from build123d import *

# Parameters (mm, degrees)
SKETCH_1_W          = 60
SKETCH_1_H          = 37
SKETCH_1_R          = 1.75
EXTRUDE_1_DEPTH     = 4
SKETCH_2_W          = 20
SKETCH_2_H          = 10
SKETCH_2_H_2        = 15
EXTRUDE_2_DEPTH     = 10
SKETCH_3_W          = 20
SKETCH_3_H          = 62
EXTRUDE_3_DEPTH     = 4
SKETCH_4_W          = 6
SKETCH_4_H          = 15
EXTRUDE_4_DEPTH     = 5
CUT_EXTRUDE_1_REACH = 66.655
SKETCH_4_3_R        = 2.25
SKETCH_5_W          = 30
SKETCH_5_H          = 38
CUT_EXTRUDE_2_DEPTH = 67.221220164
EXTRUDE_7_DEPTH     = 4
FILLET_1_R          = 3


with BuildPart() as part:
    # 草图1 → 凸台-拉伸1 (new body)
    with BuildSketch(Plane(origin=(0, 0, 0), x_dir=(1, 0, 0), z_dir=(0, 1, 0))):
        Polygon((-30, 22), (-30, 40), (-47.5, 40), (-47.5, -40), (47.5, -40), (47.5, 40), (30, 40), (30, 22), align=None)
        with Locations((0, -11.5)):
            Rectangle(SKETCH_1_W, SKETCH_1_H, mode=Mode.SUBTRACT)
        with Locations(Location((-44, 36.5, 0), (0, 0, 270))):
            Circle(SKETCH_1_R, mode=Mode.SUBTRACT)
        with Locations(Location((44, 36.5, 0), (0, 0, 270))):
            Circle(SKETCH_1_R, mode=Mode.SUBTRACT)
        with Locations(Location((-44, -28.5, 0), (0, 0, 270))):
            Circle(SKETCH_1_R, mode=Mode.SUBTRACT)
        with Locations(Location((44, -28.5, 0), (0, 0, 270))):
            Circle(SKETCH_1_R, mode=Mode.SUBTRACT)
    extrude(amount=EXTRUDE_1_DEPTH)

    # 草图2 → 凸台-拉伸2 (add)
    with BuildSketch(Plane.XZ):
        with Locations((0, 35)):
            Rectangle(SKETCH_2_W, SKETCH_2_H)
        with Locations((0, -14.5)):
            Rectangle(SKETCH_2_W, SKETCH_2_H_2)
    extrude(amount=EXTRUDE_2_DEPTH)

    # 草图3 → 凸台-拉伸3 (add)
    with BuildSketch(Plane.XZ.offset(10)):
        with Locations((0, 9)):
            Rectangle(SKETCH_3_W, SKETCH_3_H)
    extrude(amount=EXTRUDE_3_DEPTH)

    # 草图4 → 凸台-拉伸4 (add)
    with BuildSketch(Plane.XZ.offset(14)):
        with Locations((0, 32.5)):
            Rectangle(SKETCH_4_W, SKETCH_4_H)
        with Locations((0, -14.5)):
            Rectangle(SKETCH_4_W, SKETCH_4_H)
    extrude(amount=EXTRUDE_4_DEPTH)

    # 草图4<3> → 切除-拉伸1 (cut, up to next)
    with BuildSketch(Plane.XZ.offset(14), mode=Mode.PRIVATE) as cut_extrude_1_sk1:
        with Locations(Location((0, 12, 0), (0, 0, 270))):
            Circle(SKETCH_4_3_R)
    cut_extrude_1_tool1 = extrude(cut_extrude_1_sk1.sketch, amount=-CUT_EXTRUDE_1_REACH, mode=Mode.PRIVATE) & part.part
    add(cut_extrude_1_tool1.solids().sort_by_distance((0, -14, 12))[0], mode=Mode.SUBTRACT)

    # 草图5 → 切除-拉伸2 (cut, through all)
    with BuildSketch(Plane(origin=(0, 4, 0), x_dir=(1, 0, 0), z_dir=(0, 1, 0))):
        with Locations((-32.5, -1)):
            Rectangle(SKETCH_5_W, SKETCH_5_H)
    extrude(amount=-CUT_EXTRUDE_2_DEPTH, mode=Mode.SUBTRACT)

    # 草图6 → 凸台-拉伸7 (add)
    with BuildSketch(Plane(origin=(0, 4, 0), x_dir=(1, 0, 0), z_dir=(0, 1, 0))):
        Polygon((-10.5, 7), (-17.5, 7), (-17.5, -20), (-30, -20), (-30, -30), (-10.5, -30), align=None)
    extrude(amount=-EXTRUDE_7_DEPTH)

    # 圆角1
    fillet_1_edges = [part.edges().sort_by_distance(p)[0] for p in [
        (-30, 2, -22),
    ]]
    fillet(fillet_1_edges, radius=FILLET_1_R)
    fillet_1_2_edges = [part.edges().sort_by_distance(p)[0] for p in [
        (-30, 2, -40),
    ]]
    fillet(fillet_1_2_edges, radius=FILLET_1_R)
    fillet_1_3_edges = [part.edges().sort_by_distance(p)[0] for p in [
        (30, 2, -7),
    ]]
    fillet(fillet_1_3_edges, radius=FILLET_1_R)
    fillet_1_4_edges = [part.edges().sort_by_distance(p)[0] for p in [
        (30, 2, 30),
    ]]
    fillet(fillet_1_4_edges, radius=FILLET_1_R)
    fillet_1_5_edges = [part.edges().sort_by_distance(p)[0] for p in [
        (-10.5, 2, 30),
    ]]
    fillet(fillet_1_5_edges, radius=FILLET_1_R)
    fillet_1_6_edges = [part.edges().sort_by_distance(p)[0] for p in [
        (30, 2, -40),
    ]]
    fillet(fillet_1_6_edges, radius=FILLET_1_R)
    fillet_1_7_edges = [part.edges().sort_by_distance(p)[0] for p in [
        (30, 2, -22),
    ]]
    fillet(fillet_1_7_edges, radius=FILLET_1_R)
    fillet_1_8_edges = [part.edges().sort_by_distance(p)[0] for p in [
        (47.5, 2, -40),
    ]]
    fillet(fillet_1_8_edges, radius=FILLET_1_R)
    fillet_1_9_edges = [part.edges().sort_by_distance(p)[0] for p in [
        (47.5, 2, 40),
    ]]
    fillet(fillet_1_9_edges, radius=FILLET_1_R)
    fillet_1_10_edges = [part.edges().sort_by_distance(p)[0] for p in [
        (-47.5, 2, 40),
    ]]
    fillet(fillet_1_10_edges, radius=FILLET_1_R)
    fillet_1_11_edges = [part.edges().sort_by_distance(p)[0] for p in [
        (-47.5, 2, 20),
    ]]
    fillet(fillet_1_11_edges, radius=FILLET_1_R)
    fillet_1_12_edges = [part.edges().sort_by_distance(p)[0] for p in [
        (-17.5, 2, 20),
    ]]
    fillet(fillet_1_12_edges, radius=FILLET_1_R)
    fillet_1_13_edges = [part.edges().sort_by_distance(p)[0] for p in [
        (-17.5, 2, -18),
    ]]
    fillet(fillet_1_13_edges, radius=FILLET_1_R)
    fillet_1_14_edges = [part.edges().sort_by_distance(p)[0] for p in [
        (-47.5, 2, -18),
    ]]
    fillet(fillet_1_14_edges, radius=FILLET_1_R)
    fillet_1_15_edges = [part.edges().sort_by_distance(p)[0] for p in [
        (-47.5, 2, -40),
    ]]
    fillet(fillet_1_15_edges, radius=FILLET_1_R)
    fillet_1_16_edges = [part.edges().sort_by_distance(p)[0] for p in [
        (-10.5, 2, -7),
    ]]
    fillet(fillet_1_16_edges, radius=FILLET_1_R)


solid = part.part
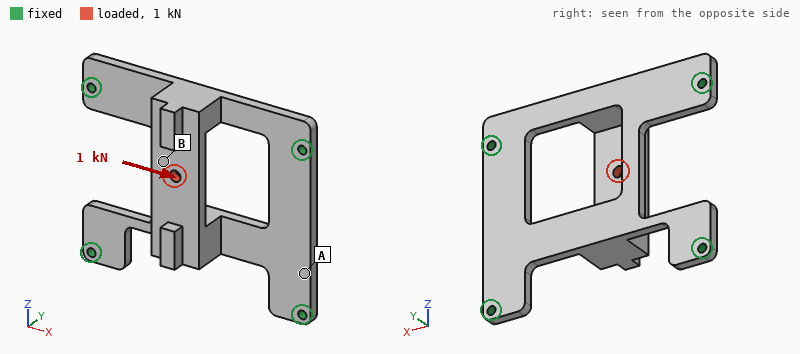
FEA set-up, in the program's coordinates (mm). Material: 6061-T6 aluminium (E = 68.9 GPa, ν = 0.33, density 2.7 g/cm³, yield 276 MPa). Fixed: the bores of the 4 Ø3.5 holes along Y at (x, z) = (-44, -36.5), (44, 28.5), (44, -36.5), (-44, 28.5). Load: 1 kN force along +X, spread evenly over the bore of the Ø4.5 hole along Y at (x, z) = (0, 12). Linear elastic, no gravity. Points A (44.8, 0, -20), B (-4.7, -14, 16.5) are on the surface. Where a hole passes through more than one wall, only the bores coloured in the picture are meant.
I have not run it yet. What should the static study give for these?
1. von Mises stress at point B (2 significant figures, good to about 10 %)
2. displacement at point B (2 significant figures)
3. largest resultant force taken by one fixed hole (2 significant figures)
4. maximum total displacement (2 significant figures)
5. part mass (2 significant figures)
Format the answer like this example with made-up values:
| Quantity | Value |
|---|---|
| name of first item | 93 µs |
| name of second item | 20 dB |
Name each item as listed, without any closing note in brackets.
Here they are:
| Quantity | Value |
|---|---|
| von Mises stress at point B | 19 MPa |
| displacement at point B | 0.089 mm |
| largest resultant force taken by one fixed hole | 370 N |
| maximum total displacement | 0.11 mm |
| part mass | 71 g |
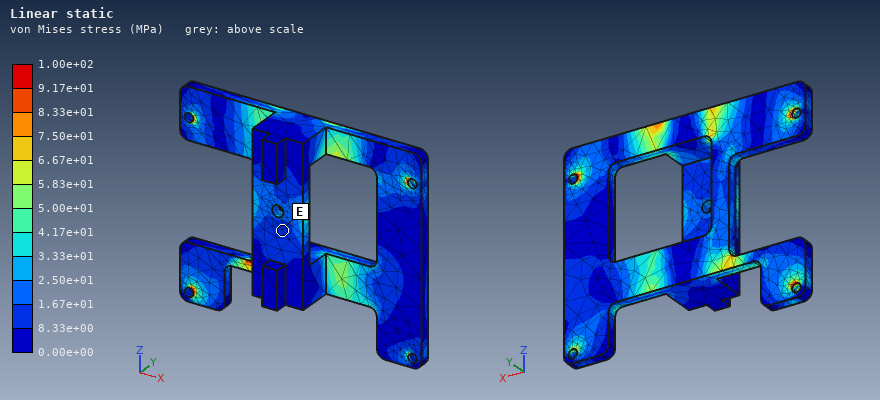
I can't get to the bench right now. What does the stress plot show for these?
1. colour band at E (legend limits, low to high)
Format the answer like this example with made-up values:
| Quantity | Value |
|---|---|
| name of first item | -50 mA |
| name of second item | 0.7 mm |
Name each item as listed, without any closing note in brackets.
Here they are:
| Quantity | Value |
|---|---|
| colour band at E | 8.33e+00 to 1.67e+01 MPa |
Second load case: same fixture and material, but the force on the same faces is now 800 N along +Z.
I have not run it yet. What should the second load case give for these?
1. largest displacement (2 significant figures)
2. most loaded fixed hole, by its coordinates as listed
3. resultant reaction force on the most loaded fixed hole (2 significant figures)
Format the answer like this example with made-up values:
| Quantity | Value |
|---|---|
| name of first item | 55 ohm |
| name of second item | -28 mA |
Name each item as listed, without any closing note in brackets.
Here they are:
| Quantity | Value |
|---|---|
| largest displacement | 0.17 mm |
| most loaded fixed hole, by its coordinates as listed | (44, -36.5) |
| resultant reaction force on the most loaded fixed hole | 400 N |
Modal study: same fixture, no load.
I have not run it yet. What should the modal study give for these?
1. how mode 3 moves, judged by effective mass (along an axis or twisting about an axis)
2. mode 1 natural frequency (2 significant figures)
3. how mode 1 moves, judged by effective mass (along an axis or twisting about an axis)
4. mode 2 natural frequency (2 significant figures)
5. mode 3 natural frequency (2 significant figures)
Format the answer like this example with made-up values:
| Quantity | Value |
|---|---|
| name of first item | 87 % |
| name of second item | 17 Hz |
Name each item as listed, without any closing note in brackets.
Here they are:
| Quantity | Value |
|---|---|
| how mode 3 moves, judged by effective mass | along X |
| mode 1 natural frequency | 1500 Hz |
| how mode 1 moves, judged by effective mass | along Y |
| mode 2 natural frequency | 1900 Hz |
| mode 3 natural frequency | 3200 Hz |
